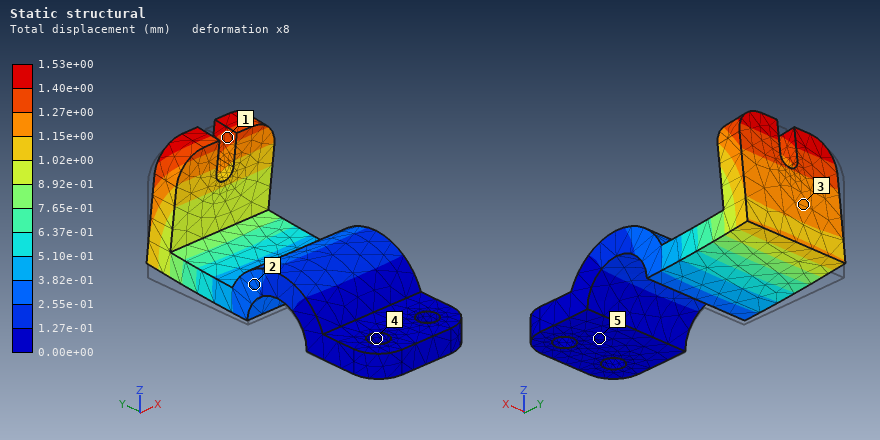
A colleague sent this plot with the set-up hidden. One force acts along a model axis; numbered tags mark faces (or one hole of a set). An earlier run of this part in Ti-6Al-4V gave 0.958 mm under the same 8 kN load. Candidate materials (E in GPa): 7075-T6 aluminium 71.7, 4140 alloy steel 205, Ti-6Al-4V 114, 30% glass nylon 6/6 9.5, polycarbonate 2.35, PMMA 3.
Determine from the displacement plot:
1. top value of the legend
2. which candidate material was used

1.53e+00 mm
7075-T6 aluminium
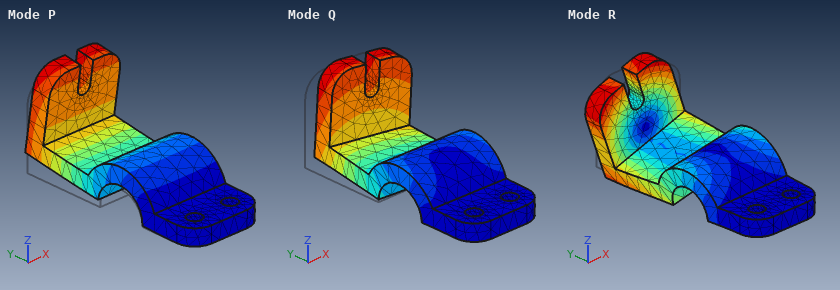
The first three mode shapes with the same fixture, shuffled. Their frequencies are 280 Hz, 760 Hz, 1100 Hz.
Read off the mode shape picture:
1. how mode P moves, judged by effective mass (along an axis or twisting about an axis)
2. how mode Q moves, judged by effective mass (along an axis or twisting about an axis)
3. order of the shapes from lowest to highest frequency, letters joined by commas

along Z
along X
P, Q, R
